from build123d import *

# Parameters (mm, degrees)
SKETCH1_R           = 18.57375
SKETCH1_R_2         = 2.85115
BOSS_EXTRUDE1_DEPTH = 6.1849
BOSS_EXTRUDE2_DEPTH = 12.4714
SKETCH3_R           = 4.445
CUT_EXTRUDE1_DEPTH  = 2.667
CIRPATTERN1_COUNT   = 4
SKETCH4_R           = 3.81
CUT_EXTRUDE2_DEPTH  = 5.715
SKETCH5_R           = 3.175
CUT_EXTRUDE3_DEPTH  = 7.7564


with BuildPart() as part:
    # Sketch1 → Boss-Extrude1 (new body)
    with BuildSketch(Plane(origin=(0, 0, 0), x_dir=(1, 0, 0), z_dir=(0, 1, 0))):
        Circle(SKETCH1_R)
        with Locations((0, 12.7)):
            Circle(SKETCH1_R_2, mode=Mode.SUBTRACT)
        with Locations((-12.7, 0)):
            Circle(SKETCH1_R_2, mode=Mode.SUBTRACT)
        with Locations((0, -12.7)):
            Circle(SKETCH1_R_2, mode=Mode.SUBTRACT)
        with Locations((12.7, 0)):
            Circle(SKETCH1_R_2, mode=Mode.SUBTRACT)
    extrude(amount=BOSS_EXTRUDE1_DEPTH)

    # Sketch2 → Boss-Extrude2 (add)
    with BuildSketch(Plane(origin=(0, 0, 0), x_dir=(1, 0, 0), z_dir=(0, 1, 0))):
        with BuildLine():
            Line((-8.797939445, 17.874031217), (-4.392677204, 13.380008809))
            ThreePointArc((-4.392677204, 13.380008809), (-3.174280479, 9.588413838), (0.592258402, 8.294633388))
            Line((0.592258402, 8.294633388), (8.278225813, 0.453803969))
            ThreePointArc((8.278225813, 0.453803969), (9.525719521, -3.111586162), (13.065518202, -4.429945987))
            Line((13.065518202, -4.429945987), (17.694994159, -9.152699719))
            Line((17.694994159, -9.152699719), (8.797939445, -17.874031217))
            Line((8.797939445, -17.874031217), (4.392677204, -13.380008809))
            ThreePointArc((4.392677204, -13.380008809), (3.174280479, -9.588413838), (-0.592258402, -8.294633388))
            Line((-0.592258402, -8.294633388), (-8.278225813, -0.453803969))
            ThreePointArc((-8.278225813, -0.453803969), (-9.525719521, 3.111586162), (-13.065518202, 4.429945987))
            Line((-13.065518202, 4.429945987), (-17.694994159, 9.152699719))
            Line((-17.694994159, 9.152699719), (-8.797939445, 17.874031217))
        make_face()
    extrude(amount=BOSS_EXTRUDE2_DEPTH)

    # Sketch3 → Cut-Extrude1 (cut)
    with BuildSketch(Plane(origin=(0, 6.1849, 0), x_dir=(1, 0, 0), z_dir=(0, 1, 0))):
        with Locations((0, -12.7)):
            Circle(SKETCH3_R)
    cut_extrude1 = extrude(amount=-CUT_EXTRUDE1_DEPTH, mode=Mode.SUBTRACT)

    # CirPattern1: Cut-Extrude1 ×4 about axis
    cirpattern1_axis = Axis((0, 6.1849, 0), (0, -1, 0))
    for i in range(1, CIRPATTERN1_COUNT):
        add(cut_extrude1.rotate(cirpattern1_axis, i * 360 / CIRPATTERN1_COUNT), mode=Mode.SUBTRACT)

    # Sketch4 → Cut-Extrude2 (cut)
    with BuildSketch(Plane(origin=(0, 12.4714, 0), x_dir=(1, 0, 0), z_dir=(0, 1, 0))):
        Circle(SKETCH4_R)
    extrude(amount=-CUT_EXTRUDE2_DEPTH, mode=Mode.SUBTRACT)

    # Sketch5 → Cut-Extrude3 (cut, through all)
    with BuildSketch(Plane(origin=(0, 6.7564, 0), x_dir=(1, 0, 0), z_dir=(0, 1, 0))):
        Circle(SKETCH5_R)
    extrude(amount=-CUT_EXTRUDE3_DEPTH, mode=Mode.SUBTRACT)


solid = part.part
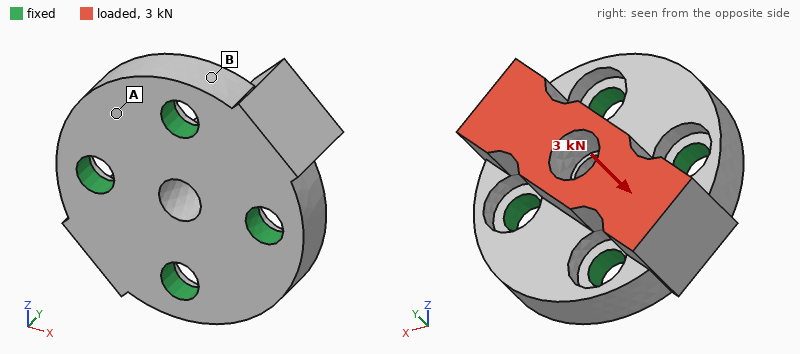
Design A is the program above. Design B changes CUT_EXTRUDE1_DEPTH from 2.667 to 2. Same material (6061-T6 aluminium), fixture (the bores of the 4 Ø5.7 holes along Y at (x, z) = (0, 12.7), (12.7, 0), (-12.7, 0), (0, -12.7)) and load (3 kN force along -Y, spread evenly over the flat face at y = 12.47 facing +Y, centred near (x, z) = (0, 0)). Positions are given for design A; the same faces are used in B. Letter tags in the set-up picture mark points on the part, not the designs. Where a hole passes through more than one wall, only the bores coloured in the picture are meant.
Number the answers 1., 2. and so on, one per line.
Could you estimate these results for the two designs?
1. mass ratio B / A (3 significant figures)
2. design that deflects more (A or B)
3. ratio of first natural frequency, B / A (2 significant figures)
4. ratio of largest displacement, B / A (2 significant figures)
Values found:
1. 1.01
2. A
3. 1.1
4. 0.92
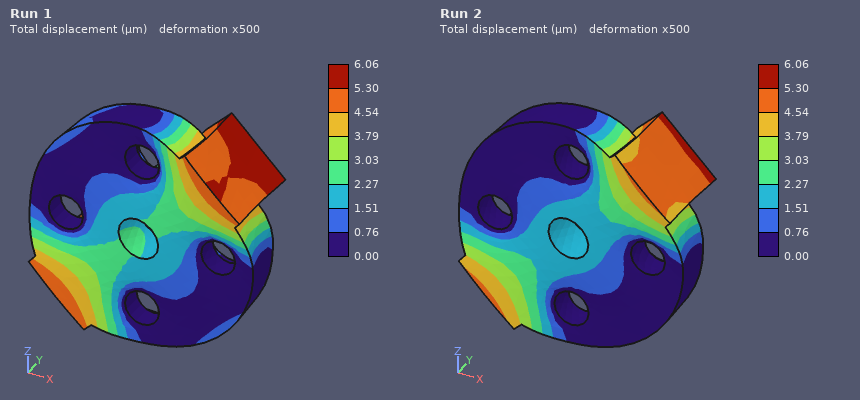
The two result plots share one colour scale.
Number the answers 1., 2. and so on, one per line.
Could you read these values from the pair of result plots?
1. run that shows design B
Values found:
1. Run 2
